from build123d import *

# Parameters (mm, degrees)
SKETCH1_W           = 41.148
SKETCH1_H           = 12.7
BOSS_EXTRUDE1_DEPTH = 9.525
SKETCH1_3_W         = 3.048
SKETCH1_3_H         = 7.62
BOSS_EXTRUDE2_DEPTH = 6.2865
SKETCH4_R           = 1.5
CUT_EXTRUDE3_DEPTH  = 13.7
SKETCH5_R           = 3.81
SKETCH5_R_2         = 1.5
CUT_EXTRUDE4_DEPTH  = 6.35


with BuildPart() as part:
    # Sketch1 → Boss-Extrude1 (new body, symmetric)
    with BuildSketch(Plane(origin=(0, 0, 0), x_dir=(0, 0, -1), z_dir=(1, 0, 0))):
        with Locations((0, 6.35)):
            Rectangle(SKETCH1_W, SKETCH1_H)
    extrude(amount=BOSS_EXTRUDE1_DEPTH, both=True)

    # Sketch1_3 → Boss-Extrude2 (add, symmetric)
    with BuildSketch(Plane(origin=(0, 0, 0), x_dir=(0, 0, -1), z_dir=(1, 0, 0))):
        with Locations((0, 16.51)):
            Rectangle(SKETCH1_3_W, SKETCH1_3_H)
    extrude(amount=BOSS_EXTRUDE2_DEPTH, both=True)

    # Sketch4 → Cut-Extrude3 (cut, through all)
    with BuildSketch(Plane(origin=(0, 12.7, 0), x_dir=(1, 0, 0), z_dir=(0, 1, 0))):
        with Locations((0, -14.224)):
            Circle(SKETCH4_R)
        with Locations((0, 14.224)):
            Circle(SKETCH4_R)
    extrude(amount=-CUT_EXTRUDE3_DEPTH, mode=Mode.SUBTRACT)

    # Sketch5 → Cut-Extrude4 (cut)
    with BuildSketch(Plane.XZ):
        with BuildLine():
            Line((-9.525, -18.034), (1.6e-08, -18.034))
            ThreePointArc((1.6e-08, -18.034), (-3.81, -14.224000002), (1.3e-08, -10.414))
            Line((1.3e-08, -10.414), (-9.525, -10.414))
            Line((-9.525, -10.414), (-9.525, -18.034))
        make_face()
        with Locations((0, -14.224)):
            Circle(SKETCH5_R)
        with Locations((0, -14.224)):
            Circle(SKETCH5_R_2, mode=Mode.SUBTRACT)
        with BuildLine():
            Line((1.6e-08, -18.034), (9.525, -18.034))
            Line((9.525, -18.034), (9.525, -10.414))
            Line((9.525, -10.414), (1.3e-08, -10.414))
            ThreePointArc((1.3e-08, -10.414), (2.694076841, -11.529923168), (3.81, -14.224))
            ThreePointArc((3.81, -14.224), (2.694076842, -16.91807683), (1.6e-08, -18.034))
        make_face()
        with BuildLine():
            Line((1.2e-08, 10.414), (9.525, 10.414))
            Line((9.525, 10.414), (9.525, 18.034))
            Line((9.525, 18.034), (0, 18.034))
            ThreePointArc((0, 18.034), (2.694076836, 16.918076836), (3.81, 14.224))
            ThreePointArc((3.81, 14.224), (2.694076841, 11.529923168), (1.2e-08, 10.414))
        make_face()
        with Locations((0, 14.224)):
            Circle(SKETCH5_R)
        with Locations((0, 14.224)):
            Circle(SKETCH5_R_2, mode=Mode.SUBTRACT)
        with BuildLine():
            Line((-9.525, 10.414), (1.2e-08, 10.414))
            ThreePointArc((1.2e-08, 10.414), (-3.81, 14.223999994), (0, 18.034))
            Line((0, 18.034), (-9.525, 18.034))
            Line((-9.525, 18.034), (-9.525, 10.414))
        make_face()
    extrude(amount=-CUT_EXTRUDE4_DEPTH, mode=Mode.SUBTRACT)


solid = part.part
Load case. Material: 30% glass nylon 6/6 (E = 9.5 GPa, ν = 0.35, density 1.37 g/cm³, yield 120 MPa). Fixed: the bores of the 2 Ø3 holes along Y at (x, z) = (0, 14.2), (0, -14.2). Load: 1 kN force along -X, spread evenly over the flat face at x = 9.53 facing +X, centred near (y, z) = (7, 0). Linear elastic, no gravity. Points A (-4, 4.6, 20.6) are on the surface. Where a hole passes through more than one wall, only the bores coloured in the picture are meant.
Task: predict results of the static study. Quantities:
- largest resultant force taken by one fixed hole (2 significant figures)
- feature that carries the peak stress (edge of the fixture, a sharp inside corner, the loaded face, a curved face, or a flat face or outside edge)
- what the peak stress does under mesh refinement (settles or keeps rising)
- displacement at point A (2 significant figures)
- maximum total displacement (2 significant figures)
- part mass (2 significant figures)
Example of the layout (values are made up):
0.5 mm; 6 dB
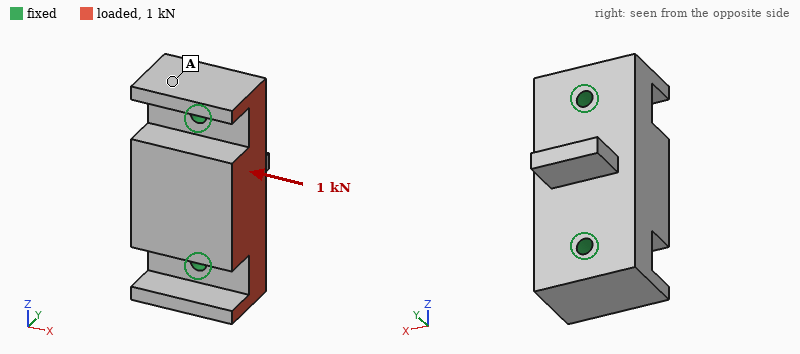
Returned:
500 N; edge of the fixture; keeps rising; 6.6 µm; 33 µm; 11 g
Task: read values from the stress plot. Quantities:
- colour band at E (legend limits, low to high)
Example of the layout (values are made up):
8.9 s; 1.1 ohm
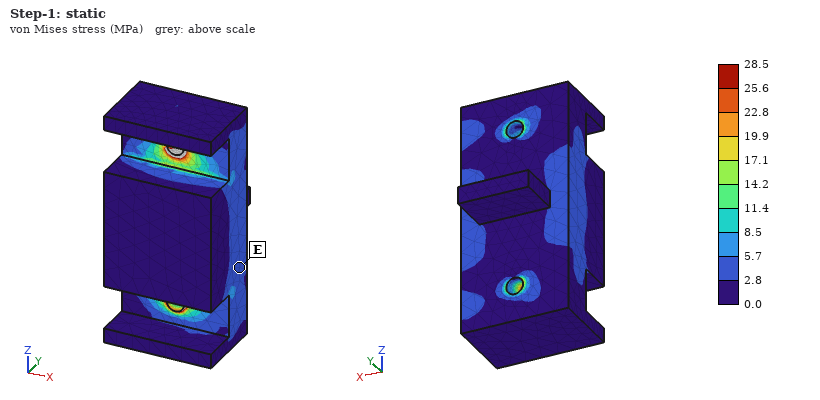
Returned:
2.8 to 5.7 MPa
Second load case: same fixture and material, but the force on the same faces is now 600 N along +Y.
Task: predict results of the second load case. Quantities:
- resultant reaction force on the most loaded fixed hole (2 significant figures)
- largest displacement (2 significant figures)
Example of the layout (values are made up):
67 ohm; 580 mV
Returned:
310 N; 61 µm
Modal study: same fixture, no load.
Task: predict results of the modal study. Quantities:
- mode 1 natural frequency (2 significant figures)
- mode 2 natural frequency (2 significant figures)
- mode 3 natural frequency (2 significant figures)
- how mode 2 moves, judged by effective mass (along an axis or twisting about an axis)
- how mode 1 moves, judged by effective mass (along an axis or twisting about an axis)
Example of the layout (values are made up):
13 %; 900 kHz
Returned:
8300 Hz; 13 kHz; 15 kHz; along Y; along X
